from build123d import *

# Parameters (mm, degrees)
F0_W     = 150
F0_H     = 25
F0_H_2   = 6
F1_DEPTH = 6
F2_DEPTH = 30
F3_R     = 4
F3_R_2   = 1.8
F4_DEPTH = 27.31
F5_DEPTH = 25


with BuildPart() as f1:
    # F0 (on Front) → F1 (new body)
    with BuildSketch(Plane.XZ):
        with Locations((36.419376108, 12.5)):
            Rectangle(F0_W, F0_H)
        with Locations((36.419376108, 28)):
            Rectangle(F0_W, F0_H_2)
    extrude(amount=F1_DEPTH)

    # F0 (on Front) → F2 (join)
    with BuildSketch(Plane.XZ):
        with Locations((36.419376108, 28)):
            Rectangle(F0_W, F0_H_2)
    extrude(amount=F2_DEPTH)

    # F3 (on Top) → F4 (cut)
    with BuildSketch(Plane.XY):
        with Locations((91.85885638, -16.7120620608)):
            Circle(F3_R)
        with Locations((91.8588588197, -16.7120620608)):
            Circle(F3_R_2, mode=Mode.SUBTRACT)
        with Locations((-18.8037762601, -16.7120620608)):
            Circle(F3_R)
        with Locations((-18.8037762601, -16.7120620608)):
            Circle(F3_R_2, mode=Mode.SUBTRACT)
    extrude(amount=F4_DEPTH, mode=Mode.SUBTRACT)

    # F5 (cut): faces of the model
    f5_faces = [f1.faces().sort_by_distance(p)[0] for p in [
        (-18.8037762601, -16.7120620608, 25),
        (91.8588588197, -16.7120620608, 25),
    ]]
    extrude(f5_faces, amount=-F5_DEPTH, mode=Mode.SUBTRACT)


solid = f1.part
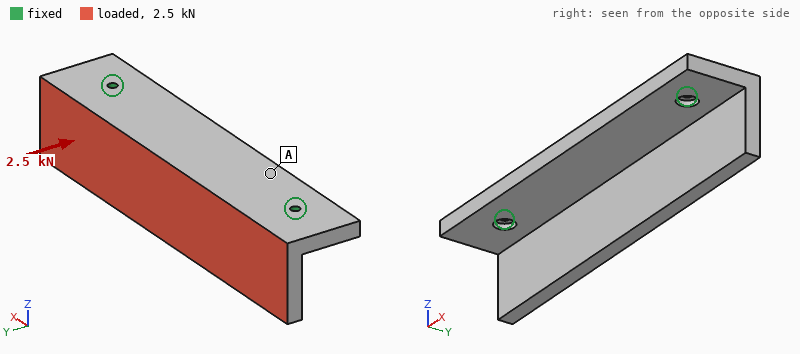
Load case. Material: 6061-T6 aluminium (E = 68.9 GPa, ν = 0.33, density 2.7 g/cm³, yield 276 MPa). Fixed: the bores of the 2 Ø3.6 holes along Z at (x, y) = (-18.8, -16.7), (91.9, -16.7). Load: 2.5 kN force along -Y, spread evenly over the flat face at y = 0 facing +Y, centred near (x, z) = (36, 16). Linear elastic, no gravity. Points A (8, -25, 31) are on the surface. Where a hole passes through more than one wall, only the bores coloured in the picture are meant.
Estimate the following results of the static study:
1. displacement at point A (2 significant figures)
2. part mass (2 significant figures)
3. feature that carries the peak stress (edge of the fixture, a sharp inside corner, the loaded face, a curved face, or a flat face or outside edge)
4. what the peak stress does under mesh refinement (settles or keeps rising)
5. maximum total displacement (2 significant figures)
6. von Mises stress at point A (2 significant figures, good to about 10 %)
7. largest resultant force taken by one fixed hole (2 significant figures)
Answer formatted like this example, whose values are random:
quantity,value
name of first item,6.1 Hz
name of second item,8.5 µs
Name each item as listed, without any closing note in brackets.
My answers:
quantity,value
displacement at point A,0.084 mm
part mass,130 g
feature that carries the peak stress,edge of the fixture
what the peak stress does under mesh refinement,keeps rising
maximum total displacement,0.38 mm
von Mises stress at point A,25 MPa
largest resultant force taken by one fixed hole,1.3 kN
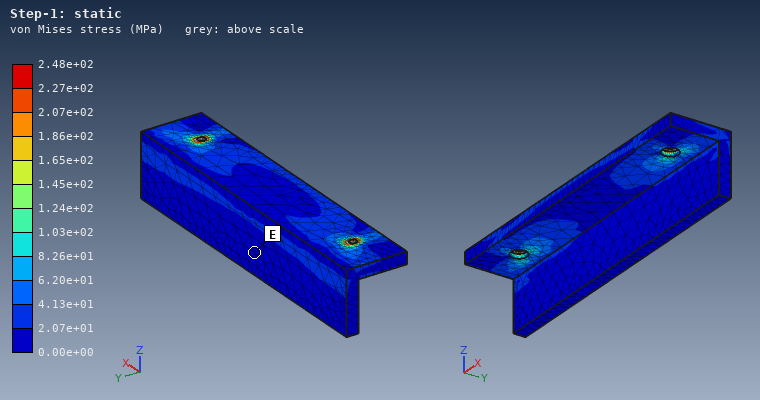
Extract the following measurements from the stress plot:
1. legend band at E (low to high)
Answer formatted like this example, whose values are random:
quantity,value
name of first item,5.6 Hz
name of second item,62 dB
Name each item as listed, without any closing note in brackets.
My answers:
quantity,value
legend band at E,0.00e+00 to 2.07e+01 MPa
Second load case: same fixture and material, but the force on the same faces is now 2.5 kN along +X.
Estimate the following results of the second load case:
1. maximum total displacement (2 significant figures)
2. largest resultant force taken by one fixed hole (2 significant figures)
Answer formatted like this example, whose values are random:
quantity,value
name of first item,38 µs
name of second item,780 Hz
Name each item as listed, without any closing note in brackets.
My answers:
quantity,value
maximum total displacement,24 µm
largest resultant force taken by one fixed hole,1.3 kN
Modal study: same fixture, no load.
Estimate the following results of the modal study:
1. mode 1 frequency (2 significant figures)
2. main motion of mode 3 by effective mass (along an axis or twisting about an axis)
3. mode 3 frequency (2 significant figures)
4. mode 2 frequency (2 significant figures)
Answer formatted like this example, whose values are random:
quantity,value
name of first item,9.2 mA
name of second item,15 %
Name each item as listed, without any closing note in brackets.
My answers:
quantity,value
mode 1 frequency,1600 Hz
main motion of mode 3 by effective mass,along Z
mode 3 frequency,3500 Hz
mode 2 frequency,2900 Hz
